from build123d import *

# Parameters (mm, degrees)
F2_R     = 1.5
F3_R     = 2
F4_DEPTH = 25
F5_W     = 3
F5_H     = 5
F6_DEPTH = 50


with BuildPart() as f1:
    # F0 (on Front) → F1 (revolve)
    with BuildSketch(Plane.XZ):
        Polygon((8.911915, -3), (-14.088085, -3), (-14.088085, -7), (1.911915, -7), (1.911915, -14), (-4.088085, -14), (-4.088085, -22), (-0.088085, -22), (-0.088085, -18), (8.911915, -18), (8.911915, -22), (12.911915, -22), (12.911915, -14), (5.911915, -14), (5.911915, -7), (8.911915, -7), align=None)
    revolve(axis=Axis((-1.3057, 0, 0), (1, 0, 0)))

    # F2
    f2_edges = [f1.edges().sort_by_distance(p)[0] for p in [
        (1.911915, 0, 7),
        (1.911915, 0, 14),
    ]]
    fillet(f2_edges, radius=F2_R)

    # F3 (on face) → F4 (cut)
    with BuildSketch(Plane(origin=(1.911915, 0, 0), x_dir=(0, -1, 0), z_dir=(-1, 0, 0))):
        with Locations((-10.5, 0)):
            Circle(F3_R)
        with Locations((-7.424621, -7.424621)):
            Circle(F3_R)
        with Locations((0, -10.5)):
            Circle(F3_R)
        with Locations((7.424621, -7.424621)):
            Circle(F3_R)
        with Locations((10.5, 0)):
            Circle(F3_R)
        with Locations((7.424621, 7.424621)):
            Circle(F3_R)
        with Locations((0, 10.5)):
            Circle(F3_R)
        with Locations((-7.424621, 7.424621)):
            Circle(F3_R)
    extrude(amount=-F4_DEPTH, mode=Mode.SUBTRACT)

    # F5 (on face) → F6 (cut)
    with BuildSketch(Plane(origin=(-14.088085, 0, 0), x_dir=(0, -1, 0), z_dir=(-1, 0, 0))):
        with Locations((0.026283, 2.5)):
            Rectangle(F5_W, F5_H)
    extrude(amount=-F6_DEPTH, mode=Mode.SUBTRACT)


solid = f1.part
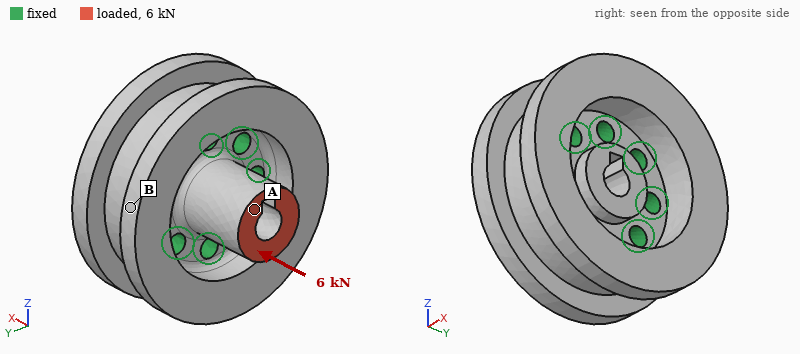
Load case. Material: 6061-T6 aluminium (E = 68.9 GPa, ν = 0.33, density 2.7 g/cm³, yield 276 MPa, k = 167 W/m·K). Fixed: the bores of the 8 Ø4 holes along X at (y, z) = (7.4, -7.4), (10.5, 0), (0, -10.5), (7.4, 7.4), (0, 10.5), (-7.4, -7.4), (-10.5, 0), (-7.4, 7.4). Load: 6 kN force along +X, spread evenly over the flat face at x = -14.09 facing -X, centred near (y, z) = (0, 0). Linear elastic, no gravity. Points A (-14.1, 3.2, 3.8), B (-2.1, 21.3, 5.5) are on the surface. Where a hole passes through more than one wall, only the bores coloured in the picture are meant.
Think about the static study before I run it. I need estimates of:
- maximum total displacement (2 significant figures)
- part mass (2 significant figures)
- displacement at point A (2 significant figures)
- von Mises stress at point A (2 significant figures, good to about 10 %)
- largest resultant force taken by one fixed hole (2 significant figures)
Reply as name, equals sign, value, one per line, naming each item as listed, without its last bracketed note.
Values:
maximum total displacement = 16 µm
part mass = 41 g
displacement at point A = 16 µm
von Mises stress at point A = 51 MPa
largest resultant force taken by one fixed hole = 850 N
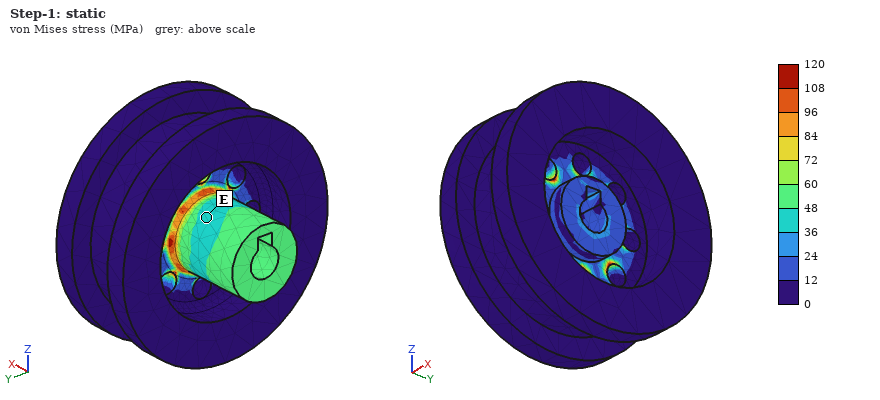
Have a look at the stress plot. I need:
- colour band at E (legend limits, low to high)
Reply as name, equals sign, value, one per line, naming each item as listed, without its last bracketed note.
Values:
colour band at E = 36 to 48 MPa
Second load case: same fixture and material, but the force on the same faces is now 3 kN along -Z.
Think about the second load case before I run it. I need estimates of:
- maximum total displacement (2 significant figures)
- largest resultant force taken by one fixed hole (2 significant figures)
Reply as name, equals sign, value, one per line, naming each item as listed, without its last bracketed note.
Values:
maximum total displacement = 82 µm
largest resultant force taken by one fixed hole = 1.7 kN
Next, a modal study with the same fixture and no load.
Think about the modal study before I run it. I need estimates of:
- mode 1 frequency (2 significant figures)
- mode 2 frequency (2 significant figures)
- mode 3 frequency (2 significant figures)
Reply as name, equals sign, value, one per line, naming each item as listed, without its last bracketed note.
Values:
mode 1 frequency = 20 kHz
mode 2 frequency = 20 kHz
mode 3 frequency = 21 kHz
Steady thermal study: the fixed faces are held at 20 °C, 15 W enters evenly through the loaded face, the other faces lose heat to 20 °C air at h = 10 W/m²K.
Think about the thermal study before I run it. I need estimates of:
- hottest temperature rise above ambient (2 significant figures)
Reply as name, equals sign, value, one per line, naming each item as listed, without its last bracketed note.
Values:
hottest temperature rise above ambient = 14 K
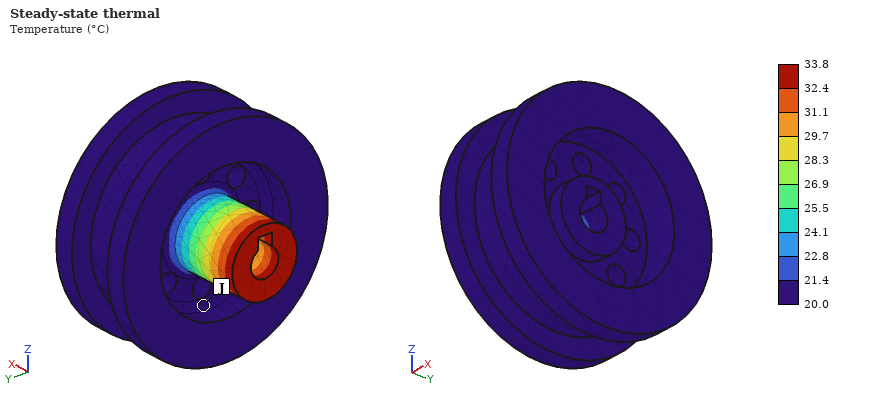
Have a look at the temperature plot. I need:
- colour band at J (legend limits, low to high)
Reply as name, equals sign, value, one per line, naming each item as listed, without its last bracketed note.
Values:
colour band at J = 20.0 to 21.4 °C
